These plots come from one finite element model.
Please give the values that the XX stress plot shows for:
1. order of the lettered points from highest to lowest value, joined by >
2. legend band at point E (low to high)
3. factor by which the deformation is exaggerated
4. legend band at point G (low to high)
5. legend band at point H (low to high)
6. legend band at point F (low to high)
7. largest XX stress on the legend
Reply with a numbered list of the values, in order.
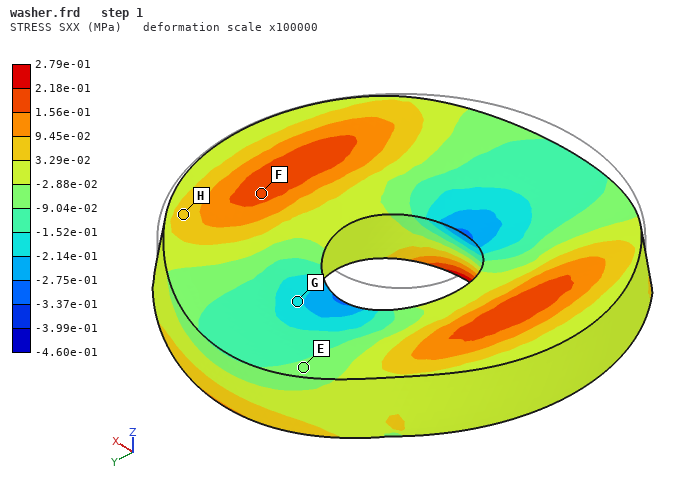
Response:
1. F > H > E > G
2. -9.04e-02 to -2.88e-02 MPa
3. 100000
4. -2.14e-01 to -1.52e-01 MPa
5. 3.29e-02 to 9.45e-02 MPa
6. 1.56e-01 to 2.18e-01 MPa
7. 2.79e-01 MPa
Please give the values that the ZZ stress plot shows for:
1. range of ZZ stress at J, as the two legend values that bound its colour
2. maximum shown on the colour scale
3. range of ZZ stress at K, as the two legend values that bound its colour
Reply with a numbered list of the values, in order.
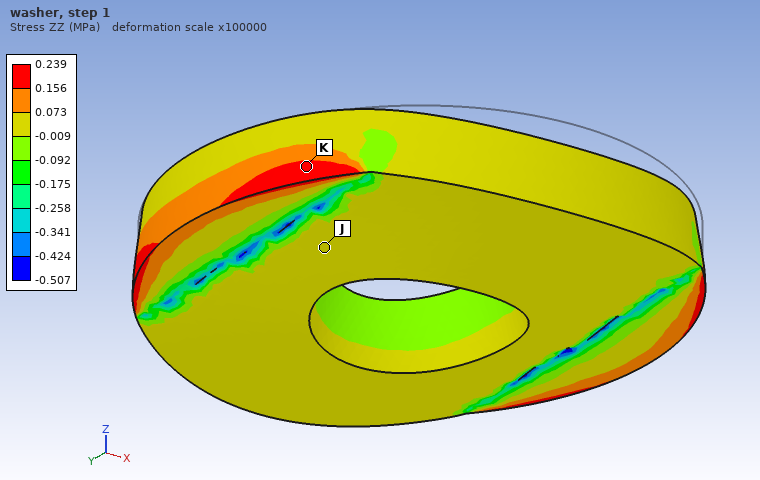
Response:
1. -0.009 to 0.073 MPa
2. 0.239 MPa
3. 0.156 to 0.239 MPa
